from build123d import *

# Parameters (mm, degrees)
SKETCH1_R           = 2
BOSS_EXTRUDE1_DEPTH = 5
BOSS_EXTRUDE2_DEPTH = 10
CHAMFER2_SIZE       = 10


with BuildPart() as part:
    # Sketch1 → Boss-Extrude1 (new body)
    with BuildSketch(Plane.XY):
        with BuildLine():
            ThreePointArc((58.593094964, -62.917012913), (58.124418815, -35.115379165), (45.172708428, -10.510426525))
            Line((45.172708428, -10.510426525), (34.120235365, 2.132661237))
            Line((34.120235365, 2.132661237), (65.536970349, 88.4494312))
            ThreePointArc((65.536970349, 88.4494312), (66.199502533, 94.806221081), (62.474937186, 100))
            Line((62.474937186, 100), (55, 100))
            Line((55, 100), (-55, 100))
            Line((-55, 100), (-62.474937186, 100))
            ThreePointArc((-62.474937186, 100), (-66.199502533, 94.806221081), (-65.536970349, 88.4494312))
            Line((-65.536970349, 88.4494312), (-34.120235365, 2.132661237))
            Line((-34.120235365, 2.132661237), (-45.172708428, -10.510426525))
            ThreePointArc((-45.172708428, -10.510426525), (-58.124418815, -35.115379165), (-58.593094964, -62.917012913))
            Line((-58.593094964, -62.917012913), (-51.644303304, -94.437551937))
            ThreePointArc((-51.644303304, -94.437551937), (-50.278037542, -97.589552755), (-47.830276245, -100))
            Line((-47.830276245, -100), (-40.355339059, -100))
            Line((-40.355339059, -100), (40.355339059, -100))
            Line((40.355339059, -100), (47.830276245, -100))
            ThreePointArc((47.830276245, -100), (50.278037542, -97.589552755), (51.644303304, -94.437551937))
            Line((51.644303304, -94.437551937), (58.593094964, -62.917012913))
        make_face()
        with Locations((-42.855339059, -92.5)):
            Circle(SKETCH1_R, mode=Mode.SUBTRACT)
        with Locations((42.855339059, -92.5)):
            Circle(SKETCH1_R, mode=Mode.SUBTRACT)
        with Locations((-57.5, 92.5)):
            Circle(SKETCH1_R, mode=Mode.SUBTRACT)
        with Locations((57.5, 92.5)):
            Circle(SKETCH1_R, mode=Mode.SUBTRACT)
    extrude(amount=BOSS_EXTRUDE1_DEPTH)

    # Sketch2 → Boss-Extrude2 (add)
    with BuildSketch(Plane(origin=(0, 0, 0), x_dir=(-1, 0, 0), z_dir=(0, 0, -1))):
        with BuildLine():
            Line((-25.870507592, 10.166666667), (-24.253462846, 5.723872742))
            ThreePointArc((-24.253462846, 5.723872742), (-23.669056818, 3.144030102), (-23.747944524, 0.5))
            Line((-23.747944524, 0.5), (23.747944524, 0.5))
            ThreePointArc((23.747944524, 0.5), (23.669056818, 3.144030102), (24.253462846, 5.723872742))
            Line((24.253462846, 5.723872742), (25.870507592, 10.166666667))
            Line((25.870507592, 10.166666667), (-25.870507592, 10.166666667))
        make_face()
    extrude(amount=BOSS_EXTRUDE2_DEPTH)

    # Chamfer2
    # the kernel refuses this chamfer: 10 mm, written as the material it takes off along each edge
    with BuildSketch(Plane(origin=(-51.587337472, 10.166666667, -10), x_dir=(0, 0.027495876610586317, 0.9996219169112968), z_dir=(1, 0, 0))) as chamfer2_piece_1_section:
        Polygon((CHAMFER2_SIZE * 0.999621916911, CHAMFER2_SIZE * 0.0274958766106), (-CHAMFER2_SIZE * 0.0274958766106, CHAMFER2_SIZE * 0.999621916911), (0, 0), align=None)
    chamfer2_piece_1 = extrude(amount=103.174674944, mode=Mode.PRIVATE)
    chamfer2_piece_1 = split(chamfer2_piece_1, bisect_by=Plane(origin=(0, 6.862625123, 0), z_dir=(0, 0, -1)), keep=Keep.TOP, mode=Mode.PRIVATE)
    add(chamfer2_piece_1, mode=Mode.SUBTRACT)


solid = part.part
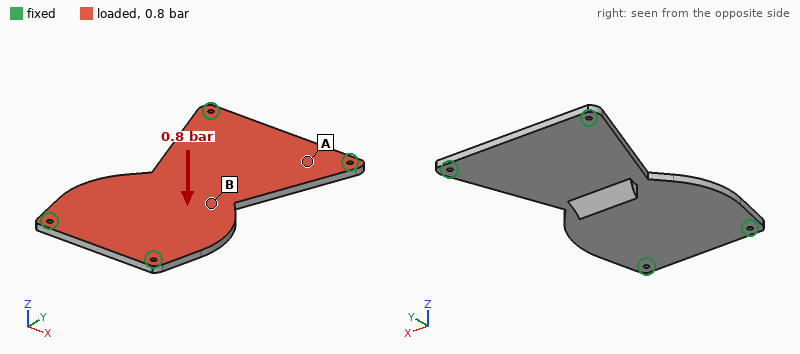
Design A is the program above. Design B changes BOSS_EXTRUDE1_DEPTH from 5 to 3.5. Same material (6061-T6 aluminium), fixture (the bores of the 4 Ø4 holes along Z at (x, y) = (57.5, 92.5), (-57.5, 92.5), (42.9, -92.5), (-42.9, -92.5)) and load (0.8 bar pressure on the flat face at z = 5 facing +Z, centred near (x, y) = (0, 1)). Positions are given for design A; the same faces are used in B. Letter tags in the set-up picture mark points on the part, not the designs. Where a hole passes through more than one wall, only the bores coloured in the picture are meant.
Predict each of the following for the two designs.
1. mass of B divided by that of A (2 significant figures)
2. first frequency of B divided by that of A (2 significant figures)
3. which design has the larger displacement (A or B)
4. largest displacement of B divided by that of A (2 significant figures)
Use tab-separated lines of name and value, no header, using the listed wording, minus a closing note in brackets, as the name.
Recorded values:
mass of B divided by that of A	0.71
first frequency of B divided by that of A	0.71
which design has the larger displacement	B
largest displacement of B divided by that of A	2.8
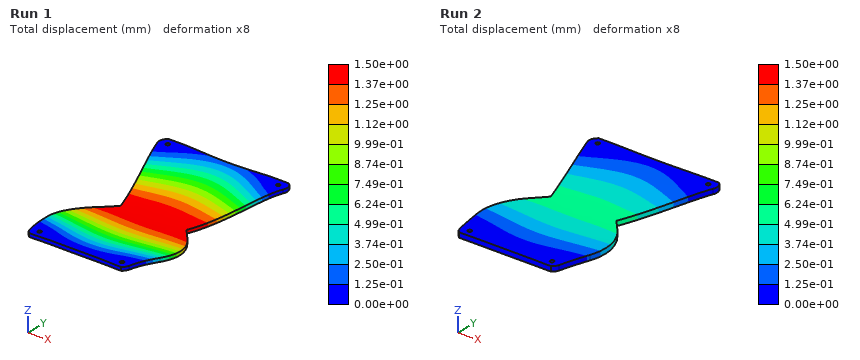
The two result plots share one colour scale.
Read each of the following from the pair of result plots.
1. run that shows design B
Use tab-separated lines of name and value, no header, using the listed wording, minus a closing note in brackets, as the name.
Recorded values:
run that shows design B	Run 1
